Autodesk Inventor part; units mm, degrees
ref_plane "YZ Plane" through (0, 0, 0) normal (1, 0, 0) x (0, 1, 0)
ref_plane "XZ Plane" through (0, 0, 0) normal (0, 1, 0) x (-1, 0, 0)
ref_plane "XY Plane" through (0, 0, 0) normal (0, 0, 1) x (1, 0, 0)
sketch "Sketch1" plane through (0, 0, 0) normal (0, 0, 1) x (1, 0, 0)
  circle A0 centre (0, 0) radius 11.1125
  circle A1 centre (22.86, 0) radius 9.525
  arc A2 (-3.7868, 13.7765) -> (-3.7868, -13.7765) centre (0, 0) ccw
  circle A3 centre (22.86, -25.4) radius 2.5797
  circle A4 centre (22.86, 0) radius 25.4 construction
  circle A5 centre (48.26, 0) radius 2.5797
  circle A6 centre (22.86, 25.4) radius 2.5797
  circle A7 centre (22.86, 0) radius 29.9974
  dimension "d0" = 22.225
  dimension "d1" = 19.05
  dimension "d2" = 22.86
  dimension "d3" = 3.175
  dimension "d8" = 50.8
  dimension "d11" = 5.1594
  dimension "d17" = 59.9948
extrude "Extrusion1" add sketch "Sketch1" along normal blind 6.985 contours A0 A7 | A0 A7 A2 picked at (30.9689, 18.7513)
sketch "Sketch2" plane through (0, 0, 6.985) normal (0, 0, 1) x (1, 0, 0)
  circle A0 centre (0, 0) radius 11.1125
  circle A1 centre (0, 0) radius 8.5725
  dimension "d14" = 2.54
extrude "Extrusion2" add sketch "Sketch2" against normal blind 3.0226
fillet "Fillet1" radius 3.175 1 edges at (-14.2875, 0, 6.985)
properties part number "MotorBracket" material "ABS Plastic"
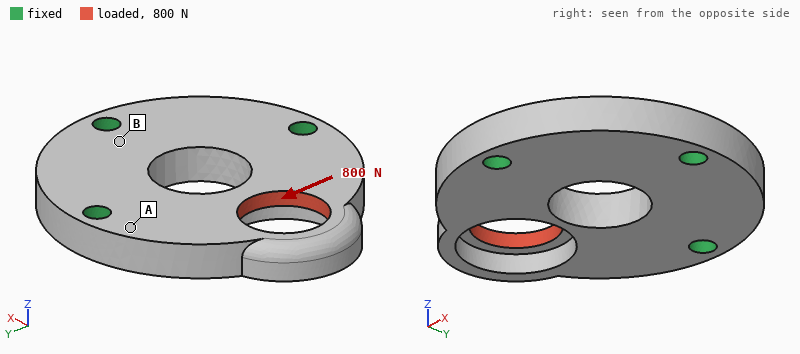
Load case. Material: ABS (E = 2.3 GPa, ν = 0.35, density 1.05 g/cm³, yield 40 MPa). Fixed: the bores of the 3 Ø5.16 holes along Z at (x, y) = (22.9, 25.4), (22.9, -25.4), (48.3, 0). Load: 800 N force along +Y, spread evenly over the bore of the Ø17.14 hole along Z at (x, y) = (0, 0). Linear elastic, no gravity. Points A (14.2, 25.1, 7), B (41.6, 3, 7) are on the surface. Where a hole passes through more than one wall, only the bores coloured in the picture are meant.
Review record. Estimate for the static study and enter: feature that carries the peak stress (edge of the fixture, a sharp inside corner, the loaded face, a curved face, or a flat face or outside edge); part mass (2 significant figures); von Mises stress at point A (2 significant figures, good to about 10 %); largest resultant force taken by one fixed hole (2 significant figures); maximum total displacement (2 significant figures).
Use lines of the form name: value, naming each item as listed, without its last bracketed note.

feature that carries the peak stress: the loaded face
part mass: 17 g
von Mises stress at point A: 5.9 MPa
largest resultant force taken by one fixed hole: 510 N
maximum total displacement: 0.35 mm
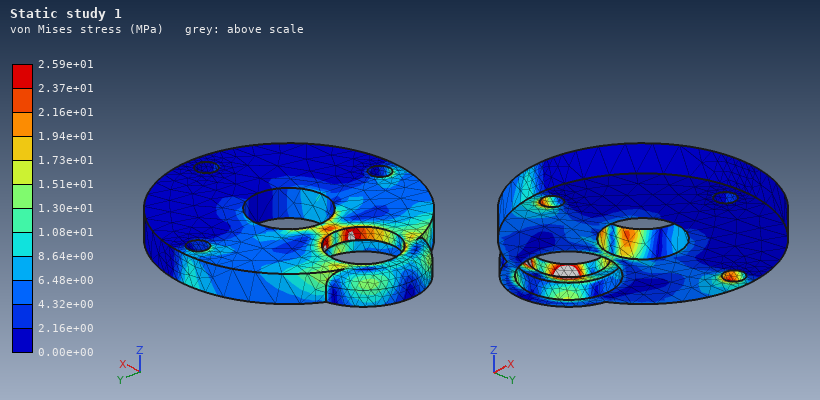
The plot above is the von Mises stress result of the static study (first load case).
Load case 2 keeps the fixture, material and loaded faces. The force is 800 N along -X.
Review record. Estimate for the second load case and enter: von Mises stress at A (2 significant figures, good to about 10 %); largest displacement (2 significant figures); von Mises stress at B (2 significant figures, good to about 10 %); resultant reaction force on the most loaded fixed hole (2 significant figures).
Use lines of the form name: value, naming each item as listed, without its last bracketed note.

von Mises stress at A: 6.3 MPa
largest displacement: 0.56 mm
von Mises stress at B: 1.8 MPa
resultant reaction force on the most loaded fixed hole: 360 N
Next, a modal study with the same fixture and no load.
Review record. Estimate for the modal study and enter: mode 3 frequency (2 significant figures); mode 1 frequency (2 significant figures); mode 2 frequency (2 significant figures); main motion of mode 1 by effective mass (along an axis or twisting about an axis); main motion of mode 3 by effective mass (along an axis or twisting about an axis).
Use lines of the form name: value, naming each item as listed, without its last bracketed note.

mode 3 frequency: 4500 Hz
mode 1 frequency: 1600 Hz
mode 2 frequency: 3400 Hz
main motion of mode 1 by effective mass: along Z
main motion of mode 3 by effective mass: along Z
